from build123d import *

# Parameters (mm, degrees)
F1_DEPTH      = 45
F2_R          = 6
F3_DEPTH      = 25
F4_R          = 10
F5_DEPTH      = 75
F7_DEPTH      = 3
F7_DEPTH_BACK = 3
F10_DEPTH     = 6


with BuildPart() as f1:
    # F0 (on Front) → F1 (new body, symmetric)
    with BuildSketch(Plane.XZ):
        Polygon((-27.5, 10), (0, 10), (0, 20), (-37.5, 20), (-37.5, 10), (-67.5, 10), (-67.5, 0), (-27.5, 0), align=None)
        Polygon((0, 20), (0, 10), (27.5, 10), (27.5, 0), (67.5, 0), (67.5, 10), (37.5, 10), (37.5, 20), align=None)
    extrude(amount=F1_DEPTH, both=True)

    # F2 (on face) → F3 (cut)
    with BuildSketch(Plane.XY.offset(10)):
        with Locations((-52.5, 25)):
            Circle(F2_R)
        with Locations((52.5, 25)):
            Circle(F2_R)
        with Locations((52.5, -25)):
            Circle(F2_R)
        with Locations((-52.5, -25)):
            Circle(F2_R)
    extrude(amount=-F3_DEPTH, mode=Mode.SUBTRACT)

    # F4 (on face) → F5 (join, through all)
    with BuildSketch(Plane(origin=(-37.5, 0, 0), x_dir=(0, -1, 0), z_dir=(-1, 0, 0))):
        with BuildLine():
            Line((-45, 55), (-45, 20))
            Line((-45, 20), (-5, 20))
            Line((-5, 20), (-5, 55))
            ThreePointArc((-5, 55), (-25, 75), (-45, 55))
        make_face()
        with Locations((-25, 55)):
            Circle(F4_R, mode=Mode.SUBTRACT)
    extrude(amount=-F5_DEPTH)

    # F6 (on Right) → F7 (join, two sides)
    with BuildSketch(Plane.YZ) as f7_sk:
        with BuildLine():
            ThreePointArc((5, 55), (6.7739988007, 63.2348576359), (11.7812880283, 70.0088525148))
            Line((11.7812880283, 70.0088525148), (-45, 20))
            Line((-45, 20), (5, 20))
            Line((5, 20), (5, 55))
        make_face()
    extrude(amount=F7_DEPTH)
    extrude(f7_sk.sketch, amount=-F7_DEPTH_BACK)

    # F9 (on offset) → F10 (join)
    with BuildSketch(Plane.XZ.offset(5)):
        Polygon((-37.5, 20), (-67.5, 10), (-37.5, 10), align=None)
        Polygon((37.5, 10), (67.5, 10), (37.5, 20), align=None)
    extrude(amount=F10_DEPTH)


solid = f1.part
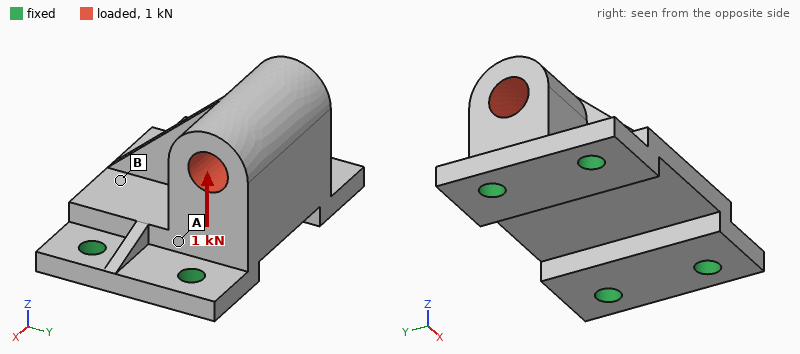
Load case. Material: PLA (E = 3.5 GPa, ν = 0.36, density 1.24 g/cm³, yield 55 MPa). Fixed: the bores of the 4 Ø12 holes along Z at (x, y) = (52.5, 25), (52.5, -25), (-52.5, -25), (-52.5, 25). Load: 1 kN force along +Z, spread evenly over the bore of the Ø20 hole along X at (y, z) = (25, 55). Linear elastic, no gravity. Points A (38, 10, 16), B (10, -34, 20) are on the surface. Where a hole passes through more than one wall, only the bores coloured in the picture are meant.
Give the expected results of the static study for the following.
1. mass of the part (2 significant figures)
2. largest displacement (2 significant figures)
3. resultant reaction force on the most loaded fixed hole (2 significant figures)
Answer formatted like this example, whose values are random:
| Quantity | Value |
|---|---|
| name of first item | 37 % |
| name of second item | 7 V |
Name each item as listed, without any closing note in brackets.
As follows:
| Quantity | Value |
|---|---|
| mass of the part | 340 g |
| largest displacement | 80 µm |
| resultant reaction force on the most loaded fixed hole | 580 N |
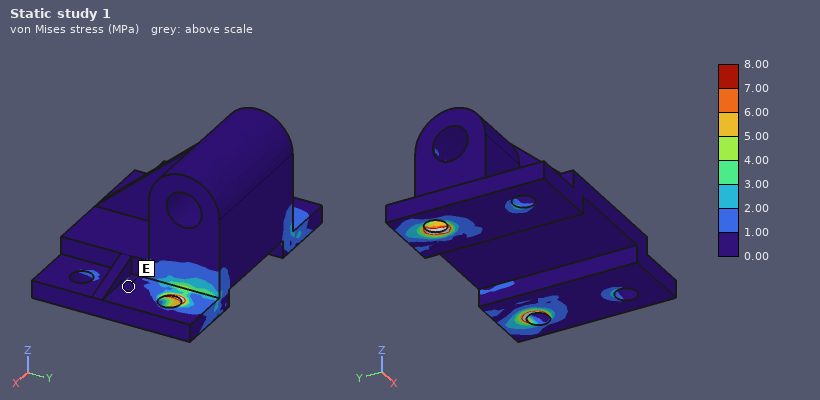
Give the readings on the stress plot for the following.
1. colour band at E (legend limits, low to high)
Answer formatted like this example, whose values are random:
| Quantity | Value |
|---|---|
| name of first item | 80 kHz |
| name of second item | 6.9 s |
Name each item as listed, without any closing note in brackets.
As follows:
| Quantity | Value |
|---|---|
| colour band at E | 0.00 to 1.00 MPa |
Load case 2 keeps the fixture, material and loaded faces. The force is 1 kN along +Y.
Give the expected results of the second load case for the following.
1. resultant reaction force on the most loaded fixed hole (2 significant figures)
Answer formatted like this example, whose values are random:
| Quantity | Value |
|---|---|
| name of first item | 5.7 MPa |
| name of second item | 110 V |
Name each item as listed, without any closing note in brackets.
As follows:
| Quantity | Value |
|---|---|
| resultant reaction force on the most loaded fixed hole | 820 N |
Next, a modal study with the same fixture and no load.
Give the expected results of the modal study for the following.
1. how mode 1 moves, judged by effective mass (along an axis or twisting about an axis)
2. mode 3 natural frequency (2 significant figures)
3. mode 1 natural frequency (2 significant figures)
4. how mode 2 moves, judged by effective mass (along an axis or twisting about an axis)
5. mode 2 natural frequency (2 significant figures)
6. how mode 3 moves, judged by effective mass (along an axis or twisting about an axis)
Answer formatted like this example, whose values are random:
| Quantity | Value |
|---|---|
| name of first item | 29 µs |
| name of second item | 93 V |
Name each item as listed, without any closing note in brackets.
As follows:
| Quantity | Value |
|---|---|
| how mode 1 moves, judged by effective mass | along Y |
| mode 3 natural frequency | 1700 Hz |
| mode 1 natural frequency | 960 Hz |
| how mode 2 moves, judged by effective mass | along X |
| mode 2 natural frequency | 1600 Hz |
| how mode 3 moves, judged by effective mass | along Z |
